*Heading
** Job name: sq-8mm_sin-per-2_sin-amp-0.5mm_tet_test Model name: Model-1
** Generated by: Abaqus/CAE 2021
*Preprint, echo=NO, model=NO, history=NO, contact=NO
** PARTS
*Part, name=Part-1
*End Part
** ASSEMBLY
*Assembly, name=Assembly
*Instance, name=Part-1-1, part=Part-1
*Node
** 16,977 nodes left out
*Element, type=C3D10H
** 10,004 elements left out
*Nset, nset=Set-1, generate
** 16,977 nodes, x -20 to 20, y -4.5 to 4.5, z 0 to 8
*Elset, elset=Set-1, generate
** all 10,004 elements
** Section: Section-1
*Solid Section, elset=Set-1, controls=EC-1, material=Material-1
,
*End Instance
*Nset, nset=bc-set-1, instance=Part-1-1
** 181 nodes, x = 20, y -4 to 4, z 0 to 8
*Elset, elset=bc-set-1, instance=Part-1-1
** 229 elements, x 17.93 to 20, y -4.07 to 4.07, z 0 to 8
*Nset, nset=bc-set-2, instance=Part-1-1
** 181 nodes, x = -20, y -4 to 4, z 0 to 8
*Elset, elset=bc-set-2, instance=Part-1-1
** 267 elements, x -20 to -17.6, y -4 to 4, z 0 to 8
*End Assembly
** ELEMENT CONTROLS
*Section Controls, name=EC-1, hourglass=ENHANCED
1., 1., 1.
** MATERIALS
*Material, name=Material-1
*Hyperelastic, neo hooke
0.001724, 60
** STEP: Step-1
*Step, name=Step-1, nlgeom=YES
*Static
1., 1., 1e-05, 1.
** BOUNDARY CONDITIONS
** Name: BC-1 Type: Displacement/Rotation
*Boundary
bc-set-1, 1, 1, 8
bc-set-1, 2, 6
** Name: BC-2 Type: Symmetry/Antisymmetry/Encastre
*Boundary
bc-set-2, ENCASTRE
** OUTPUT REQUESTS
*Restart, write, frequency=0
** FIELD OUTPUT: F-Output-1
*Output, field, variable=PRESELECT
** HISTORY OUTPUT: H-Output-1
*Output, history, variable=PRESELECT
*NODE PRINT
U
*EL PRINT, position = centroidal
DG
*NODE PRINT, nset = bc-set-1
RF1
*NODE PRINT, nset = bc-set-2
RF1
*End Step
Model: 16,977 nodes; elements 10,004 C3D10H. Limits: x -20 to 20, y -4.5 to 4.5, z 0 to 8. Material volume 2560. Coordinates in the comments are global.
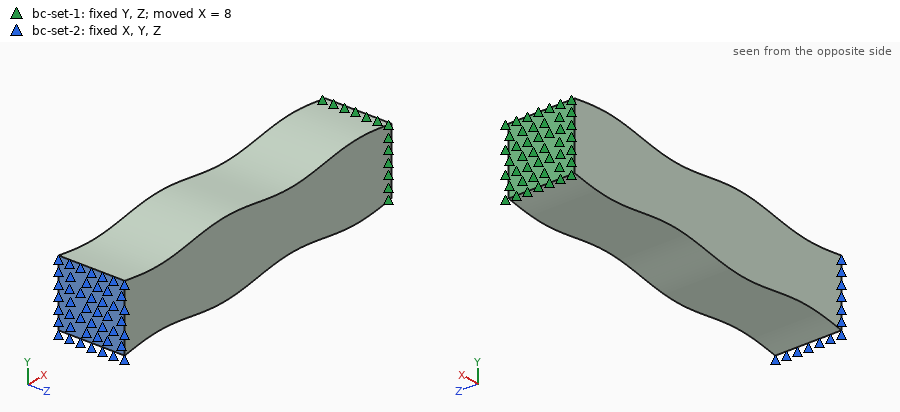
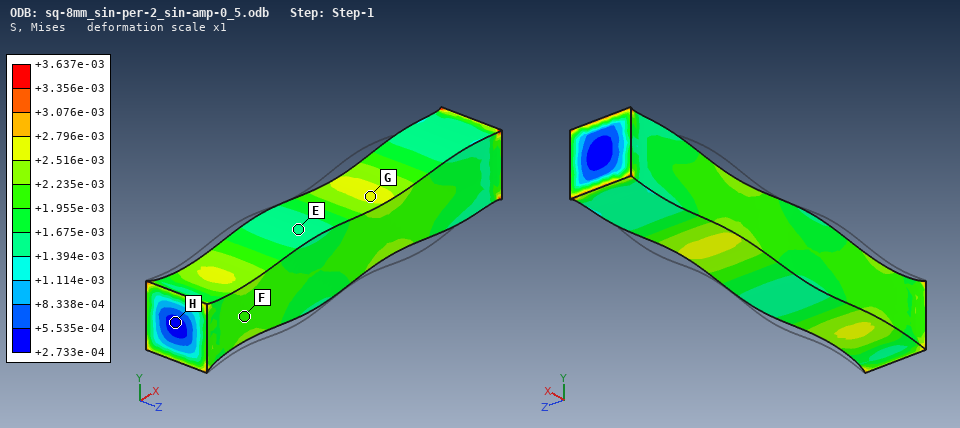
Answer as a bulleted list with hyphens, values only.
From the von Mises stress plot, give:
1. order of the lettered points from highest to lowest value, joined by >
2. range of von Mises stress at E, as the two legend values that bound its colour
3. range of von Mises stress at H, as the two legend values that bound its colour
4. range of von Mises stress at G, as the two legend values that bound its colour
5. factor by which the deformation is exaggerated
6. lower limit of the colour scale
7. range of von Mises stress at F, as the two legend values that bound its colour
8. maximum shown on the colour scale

- G > F > E > H
- +1.394e-03 to +1.675e-03
- +2.733e-04 to +5.535e-04
- +2.516e-03 to +2.796e-03
- 1
- +2.733e-04
- +1.955e-03 to +2.235e-03
- +3.637e-03
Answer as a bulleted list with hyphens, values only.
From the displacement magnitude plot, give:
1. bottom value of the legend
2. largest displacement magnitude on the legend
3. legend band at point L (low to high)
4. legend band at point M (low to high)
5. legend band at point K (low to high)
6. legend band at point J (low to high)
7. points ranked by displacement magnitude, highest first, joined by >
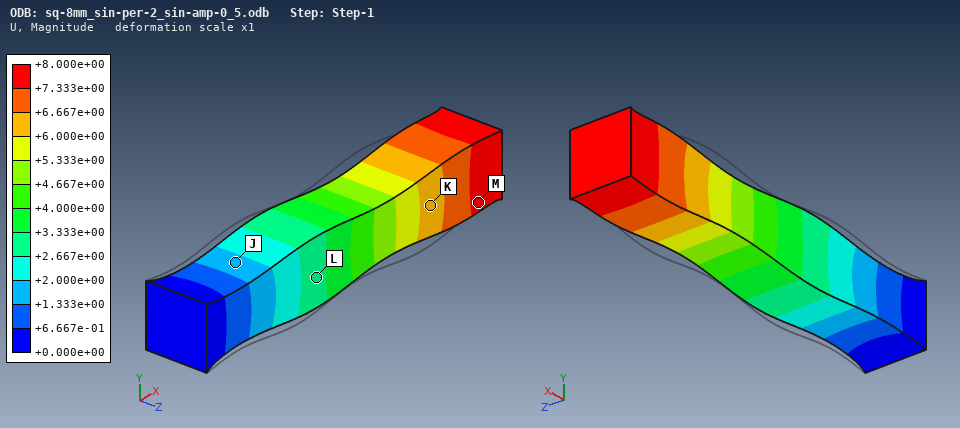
- +0.000e+00
- +8.000e+00
- +2.667e+00 to +3.333e+00
- +7.333e+00 to +8.000e+00
- +6.000e+00 to +6.667e+00
- +1.333e+00 to +2.000e+00
- M > K > L > J
